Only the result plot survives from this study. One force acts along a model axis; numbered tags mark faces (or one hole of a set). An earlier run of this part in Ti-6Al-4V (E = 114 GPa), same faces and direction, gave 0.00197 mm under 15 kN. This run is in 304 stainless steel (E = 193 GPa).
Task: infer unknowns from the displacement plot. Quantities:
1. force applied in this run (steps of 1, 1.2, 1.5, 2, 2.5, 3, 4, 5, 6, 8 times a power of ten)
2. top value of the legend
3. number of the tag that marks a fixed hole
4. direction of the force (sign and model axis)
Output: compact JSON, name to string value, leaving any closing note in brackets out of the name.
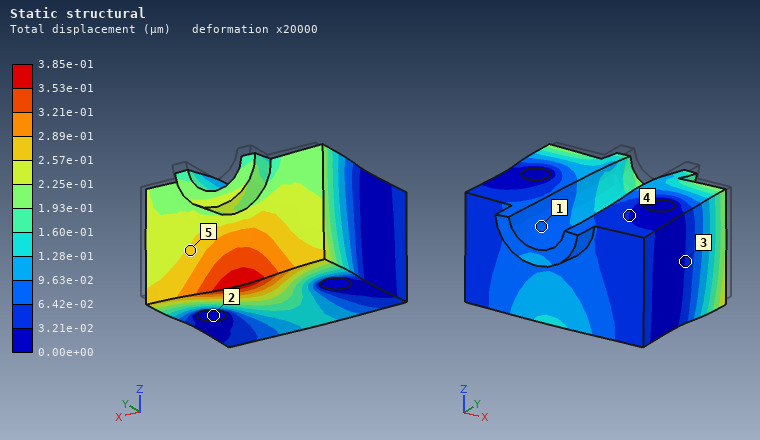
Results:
{"force applied in this run": "5 kN", "top value of the legend": "3.85e-01 µm", "number of the tag that marks a fixed hole": "2", "direction of the force": "-Y"}
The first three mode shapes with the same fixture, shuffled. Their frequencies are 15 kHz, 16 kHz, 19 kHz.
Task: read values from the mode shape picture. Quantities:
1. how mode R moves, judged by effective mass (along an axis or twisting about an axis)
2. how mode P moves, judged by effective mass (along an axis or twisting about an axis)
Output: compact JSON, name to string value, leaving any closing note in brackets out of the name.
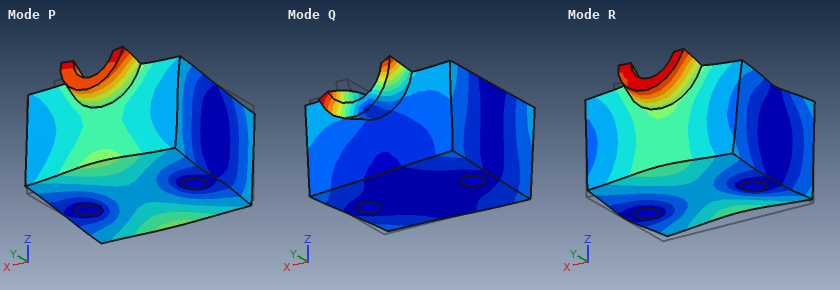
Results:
{"how mode R moves, judged by effective mass": "along Z", "how mode P moves, judged by effective mass": "twisting about X"}
